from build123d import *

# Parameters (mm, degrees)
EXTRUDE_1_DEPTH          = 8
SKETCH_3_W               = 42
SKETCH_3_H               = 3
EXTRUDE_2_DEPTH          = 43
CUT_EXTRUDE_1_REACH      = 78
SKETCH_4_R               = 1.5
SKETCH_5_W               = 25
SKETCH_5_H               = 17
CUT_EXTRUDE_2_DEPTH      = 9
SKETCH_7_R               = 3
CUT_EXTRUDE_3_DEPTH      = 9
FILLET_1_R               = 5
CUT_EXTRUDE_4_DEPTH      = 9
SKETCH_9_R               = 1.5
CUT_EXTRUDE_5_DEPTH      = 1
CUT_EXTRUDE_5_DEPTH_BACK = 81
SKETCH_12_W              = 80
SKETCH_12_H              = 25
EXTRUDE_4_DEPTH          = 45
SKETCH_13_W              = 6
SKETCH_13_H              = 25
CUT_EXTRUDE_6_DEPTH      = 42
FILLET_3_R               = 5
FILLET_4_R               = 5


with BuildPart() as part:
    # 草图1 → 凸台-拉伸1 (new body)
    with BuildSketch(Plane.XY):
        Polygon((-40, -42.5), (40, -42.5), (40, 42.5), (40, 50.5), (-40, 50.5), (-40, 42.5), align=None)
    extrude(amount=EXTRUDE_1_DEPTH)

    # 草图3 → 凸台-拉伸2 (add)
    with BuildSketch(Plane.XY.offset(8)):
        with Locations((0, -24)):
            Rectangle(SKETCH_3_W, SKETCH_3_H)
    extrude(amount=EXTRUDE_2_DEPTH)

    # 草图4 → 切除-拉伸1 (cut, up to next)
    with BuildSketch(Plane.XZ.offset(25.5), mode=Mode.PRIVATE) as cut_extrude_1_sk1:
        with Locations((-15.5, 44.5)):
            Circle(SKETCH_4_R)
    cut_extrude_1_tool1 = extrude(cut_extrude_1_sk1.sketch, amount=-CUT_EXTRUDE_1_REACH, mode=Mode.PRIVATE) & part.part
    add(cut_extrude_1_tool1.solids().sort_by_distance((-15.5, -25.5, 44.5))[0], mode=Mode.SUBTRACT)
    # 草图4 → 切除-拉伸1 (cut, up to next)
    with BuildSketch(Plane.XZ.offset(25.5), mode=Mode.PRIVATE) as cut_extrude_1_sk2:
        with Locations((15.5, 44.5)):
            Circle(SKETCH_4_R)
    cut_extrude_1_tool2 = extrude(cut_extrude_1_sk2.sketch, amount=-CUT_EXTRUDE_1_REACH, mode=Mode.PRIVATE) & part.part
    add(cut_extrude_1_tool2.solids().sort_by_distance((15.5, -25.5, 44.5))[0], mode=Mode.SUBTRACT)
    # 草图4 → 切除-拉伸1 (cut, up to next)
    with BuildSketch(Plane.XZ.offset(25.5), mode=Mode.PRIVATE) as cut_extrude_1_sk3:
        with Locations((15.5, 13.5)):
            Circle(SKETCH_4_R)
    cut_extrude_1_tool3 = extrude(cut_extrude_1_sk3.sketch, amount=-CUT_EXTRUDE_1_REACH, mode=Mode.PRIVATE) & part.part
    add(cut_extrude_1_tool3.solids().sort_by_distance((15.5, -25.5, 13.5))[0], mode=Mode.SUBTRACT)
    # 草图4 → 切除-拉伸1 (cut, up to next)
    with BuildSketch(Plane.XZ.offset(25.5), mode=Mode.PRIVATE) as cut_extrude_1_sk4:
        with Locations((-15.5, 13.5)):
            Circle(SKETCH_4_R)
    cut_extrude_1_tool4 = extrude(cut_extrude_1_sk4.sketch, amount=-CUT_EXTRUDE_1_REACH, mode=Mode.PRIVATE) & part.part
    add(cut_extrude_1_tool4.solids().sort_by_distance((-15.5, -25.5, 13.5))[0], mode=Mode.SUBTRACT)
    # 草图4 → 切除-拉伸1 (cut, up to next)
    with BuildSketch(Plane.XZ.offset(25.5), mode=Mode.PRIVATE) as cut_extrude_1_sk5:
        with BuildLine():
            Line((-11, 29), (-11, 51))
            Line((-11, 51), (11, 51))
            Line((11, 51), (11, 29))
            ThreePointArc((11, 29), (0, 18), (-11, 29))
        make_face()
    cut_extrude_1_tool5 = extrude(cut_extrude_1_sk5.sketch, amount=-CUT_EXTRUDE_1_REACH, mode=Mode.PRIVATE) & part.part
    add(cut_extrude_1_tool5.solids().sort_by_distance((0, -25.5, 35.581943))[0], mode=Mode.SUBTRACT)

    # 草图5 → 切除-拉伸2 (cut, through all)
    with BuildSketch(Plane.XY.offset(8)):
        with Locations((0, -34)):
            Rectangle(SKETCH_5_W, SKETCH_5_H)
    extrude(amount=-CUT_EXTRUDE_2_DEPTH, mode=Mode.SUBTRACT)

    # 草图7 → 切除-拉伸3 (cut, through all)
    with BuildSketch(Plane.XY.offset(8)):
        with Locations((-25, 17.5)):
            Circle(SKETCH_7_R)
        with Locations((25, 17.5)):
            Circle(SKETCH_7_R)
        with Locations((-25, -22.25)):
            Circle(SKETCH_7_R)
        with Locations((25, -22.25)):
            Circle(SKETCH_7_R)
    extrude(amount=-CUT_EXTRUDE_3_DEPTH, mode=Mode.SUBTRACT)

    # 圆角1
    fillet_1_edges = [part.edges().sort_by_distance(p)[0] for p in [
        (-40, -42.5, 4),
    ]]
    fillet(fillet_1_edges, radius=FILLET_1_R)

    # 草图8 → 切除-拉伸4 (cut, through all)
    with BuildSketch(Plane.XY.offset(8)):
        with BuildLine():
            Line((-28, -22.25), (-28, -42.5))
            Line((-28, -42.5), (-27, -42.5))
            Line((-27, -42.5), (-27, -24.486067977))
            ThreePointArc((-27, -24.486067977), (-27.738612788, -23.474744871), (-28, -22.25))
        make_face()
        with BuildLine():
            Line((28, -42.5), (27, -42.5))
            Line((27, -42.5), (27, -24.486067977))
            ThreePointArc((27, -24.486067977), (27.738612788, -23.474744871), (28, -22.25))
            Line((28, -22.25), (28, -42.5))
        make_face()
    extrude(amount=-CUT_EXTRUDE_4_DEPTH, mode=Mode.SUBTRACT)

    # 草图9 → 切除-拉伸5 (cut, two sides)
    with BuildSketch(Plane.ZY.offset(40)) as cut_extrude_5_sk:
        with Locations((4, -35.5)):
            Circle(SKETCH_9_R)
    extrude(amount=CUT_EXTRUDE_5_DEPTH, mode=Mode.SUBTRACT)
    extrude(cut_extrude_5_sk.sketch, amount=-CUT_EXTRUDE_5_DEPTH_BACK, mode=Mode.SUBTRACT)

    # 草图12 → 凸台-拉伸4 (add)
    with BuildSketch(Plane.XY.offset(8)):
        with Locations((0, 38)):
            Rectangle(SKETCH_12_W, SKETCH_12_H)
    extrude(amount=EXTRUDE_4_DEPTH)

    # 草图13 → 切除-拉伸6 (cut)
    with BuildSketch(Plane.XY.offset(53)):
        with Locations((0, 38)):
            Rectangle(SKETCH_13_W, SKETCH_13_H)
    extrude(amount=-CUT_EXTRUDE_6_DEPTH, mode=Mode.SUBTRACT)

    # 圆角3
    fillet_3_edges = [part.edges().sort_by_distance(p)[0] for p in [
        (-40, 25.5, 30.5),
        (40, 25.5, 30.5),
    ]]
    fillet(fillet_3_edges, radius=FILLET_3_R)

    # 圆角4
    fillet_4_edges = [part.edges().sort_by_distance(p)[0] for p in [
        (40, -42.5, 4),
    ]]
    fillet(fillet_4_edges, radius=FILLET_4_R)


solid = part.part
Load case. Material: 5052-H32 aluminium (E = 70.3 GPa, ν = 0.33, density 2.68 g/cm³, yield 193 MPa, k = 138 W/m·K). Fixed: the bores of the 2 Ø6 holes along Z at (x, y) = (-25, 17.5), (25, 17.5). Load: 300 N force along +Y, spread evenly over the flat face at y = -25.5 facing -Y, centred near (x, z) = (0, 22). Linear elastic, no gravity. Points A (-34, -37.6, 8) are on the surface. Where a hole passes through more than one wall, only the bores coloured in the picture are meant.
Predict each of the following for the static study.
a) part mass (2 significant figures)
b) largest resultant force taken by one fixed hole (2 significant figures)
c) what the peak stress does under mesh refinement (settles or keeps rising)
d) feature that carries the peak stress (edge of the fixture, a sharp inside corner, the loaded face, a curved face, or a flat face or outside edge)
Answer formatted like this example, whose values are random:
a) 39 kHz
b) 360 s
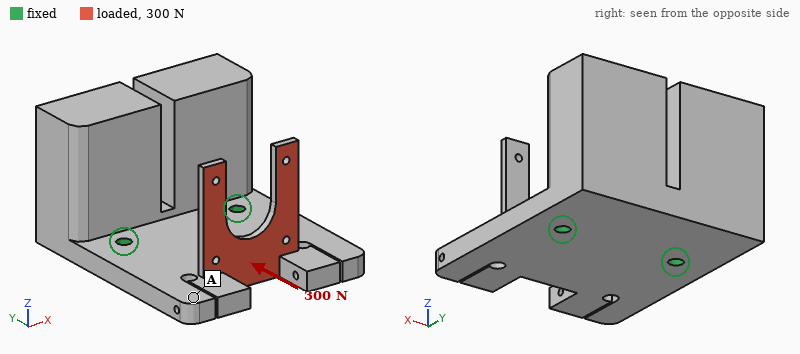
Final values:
a) 380 g
b) 150 N
c) keeps rising
d) a sharp inside corner
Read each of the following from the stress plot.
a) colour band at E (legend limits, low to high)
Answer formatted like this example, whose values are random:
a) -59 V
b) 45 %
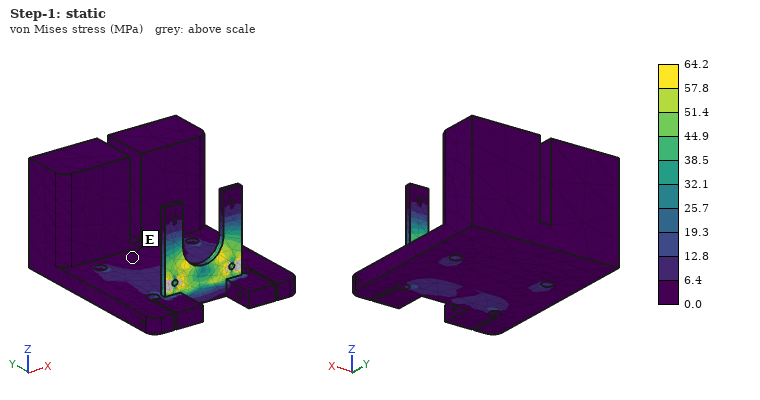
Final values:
a) 0.0 to 6.4 MPa
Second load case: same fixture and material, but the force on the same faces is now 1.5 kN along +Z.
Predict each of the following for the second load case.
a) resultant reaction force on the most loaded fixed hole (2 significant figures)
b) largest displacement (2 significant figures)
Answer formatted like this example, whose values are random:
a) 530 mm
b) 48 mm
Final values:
a) 750 N
b) 0.61 mm
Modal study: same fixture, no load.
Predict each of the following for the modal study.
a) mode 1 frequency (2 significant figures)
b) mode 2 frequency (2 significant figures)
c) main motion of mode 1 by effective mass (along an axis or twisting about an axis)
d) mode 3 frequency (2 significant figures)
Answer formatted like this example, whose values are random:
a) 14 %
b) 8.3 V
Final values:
a) 1200 Hz
b) 1500 Hz
c) along Y
d) 1600 Hz
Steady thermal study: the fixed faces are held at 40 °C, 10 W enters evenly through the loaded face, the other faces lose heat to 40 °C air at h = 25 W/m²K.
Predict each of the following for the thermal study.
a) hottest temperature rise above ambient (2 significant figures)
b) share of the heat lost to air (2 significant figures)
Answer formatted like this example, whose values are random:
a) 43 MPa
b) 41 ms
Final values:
a) 19 K
b) 17 %
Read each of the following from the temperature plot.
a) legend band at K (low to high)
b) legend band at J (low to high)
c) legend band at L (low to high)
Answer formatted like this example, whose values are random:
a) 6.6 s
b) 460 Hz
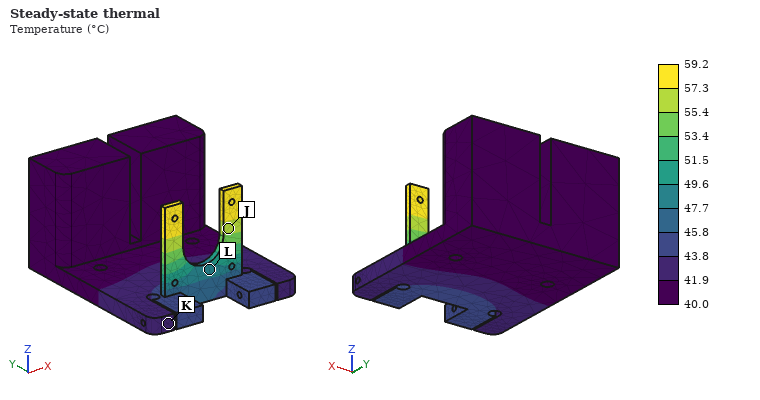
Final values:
a) 41.9 to 43.8 °C
b) 55.4 to 57.3 °C
c) 47.7 to 49.6 °C
